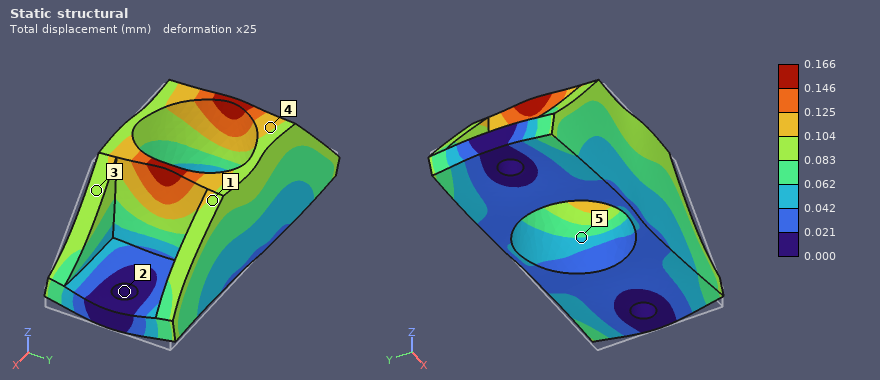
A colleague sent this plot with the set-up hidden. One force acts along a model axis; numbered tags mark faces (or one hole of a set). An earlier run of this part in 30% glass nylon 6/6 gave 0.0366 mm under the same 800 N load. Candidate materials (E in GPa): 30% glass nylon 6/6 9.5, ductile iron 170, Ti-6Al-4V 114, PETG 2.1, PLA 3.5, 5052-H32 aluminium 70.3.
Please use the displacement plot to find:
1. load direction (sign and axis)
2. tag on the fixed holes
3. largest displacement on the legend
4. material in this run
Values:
-X
2
0.166 mm
PETG
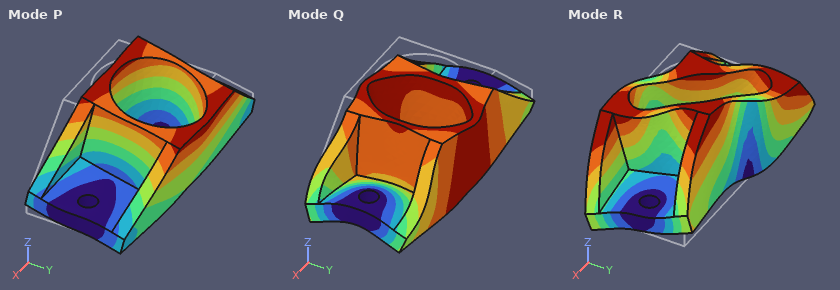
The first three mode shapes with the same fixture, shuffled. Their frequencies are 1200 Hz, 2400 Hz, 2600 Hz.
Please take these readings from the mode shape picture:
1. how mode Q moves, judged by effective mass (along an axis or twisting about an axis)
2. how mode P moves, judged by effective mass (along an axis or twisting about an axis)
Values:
along Z
along Y
